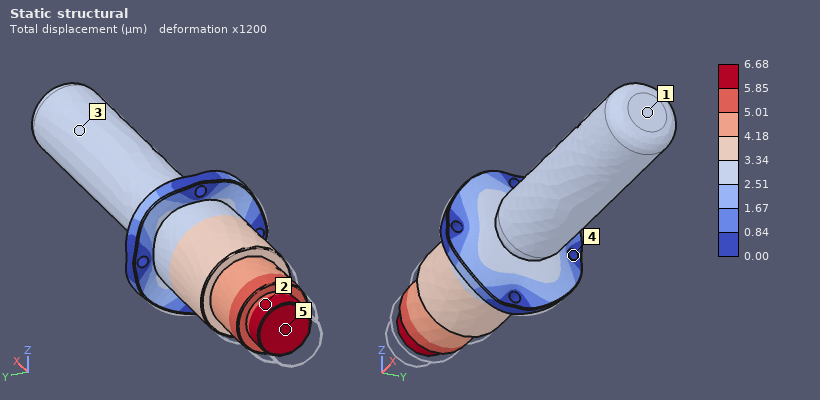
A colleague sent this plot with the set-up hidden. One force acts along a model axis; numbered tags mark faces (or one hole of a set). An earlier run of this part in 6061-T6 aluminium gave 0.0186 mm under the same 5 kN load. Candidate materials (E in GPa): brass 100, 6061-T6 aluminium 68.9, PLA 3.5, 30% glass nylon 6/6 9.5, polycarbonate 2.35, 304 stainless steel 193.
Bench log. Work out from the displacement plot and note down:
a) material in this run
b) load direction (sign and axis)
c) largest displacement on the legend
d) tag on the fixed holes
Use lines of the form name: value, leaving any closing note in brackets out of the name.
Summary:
material in this run: 304 stainless steel
load direction: +X
largest displacement on the legend: 6.68 µm
tag on the fixed holes: 4
